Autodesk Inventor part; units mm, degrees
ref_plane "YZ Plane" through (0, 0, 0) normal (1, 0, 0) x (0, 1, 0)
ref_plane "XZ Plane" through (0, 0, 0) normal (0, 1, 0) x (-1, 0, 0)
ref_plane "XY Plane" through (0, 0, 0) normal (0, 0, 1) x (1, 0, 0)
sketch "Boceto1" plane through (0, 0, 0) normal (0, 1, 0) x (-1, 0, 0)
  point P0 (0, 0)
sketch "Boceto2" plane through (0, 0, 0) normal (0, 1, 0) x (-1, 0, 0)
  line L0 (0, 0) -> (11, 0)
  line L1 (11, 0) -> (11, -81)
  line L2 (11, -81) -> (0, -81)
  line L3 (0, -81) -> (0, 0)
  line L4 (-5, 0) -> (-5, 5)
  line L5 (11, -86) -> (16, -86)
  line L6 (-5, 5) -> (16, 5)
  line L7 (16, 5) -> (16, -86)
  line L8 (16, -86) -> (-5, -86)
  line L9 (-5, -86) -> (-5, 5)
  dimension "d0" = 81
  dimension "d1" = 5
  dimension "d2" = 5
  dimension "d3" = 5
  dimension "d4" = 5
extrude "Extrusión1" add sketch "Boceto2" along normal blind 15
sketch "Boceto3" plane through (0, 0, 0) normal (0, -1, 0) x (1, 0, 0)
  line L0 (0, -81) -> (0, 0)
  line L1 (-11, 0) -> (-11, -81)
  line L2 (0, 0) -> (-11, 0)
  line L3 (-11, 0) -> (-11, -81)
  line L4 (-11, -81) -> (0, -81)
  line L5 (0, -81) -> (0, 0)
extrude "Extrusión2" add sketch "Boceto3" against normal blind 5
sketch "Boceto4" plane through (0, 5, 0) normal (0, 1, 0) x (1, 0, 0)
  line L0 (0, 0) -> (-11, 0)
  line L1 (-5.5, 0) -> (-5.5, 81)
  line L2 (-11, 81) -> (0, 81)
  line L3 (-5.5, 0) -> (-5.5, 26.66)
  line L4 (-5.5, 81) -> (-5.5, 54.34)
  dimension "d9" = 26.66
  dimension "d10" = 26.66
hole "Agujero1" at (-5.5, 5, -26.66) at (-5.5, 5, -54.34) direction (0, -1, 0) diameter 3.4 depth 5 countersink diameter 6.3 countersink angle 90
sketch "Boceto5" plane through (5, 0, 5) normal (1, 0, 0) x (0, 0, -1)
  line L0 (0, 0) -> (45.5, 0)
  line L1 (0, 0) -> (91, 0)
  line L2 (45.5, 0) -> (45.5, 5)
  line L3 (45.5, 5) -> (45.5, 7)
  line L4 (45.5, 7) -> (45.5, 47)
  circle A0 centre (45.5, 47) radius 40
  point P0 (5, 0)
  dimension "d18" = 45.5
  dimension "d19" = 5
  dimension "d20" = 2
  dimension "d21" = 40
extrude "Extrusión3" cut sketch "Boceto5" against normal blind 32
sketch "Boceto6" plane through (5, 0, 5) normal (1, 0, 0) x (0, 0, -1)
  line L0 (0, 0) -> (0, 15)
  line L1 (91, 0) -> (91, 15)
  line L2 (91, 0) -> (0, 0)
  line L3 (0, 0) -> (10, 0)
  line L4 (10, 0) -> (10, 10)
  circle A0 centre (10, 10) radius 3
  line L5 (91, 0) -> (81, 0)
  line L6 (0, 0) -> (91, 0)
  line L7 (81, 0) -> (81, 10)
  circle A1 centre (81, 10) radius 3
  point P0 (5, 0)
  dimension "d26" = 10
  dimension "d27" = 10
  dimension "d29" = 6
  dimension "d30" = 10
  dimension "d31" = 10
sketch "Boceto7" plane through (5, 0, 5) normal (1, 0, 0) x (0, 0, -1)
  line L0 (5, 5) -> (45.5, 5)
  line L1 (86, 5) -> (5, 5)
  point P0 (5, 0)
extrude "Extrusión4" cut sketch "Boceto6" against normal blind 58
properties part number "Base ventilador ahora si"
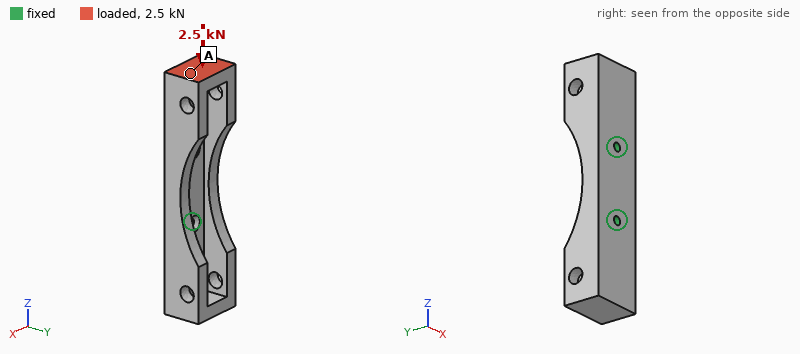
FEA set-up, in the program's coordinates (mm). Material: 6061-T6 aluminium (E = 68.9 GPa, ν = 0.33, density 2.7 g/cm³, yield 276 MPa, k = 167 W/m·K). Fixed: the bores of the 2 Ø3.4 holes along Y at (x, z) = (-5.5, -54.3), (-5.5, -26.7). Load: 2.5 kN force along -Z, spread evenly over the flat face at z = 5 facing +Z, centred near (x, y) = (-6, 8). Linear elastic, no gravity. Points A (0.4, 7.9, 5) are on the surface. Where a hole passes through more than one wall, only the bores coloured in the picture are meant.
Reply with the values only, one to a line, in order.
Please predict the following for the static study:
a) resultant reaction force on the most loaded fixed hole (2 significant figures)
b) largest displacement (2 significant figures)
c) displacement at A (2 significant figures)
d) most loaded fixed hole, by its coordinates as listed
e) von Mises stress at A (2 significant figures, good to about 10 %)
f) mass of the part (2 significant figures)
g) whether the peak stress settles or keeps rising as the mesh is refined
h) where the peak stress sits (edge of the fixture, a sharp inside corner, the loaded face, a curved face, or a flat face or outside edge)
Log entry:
1.5 kN
98 µm
88 µm
(-5.5, -26.7)
11 MPa
44 g
keeps rising
edge of the fixture
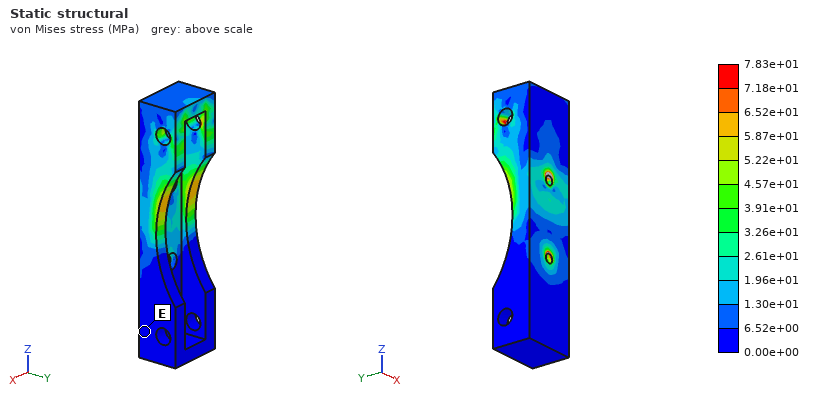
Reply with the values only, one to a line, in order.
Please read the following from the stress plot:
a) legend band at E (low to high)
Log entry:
0.00e+00 to 6.52e+00 MPa
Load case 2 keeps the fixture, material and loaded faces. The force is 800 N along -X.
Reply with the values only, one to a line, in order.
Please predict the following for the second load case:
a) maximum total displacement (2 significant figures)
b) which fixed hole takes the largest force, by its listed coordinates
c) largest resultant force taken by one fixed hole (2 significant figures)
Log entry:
0.10 mm
(-5.5, -26.7)
1.6 kN
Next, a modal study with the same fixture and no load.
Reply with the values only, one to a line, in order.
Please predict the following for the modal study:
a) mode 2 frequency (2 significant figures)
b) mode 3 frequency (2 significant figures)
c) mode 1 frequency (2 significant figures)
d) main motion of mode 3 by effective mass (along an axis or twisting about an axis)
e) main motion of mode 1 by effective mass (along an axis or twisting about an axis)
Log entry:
4100 Hz
5100 Hz
3700 Hz
along X
along Y
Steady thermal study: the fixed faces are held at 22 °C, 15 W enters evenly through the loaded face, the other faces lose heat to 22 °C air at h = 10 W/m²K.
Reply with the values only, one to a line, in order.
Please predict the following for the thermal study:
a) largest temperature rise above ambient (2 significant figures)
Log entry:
20 K
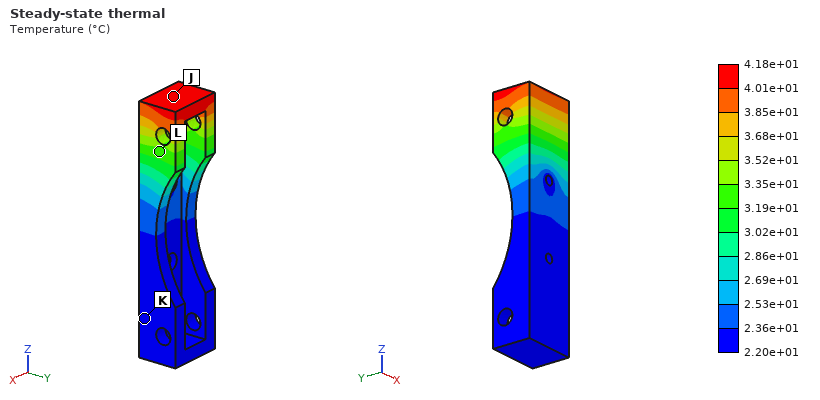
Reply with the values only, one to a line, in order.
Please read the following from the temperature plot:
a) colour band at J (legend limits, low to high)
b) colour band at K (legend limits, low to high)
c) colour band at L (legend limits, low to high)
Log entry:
4.01e+01 to 4.18e+01 °C
2.20e+01 to 2.36e+01 °C
3.19e+01 to 3.35e+01 °C
